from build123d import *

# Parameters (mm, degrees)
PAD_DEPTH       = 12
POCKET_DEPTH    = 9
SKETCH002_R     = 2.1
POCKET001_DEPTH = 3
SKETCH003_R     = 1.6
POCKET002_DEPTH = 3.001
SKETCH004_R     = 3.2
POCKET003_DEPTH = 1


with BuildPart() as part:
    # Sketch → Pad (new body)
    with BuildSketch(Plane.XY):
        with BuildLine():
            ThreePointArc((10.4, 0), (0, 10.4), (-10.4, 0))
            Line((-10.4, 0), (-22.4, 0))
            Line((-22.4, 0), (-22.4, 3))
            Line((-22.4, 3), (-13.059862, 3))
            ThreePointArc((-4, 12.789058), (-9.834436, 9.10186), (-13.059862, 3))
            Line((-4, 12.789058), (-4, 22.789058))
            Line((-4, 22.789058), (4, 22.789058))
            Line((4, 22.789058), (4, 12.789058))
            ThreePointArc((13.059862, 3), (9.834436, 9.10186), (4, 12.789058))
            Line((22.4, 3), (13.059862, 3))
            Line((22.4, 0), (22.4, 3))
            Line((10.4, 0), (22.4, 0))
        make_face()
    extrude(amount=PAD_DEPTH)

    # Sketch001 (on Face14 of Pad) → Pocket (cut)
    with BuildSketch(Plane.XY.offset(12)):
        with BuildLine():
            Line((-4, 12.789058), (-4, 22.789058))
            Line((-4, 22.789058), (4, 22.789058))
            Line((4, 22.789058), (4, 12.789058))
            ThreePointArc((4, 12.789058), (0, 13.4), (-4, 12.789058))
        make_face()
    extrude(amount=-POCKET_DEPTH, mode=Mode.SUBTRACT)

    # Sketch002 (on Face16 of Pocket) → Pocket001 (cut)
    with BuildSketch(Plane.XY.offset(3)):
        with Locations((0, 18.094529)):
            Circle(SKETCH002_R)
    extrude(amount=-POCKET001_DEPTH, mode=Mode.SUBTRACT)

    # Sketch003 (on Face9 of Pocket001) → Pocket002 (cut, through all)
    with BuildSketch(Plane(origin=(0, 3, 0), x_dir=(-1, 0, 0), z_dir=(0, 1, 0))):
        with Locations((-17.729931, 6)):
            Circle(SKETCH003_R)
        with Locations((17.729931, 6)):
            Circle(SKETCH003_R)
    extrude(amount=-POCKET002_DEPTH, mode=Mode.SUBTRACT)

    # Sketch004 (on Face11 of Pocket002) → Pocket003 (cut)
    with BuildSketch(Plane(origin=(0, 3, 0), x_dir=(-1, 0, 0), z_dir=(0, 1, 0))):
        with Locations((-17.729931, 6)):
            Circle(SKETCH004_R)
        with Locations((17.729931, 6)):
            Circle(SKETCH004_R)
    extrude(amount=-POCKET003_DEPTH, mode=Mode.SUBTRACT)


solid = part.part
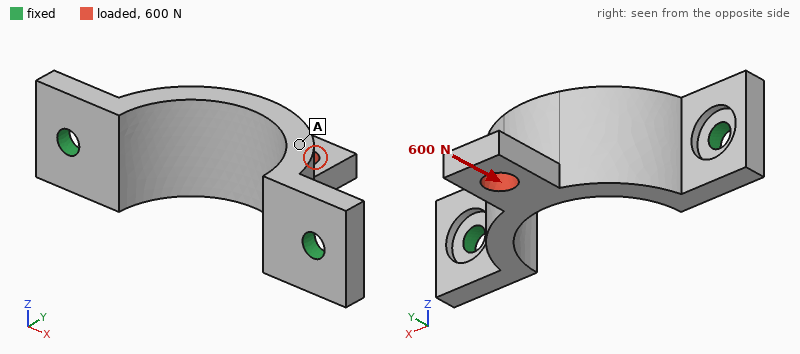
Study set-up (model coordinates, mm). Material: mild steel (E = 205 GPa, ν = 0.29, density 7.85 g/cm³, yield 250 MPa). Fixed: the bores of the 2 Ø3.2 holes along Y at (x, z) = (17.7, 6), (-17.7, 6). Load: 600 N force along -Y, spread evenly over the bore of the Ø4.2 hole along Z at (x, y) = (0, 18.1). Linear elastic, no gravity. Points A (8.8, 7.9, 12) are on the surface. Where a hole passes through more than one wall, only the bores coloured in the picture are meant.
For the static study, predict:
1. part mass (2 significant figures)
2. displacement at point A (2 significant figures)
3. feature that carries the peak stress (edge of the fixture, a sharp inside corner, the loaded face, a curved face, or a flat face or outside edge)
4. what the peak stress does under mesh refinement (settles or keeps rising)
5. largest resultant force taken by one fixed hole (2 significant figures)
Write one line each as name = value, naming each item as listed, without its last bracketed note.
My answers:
part mass = 16 g
displacement at point A = 11 µm
feature that carries the peak stress = edge of the fixture
what the peak stress does under mesh refinement = keeps rising
largest resultant force taken by one fixed hole = 430 N
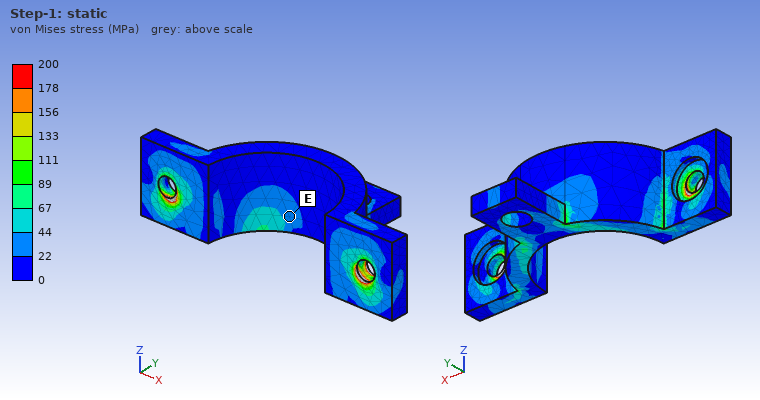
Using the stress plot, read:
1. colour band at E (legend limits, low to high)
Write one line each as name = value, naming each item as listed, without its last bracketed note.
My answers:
colour band at E = 22 to 44 MPa
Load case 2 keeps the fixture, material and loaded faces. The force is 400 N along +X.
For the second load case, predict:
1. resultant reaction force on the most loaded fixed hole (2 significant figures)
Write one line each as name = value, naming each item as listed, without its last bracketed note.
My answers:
resultant reaction force on the most loaded fixed hole = 310 N
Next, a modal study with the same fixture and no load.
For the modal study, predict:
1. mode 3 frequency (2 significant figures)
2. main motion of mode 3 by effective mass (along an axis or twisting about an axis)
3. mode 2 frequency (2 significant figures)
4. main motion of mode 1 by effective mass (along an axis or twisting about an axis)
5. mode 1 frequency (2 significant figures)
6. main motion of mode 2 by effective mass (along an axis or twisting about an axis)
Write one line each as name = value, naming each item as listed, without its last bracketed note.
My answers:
mode 3 frequency = 20 kHz
main motion of mode 3 by effective mass = along Y
mode 2 frequency = 16 kHz
main motion of mode 1 by effective mass = along Z
mode 1 frequency = 6100 Hz
main motion of mode 2 by effective mass = along X
